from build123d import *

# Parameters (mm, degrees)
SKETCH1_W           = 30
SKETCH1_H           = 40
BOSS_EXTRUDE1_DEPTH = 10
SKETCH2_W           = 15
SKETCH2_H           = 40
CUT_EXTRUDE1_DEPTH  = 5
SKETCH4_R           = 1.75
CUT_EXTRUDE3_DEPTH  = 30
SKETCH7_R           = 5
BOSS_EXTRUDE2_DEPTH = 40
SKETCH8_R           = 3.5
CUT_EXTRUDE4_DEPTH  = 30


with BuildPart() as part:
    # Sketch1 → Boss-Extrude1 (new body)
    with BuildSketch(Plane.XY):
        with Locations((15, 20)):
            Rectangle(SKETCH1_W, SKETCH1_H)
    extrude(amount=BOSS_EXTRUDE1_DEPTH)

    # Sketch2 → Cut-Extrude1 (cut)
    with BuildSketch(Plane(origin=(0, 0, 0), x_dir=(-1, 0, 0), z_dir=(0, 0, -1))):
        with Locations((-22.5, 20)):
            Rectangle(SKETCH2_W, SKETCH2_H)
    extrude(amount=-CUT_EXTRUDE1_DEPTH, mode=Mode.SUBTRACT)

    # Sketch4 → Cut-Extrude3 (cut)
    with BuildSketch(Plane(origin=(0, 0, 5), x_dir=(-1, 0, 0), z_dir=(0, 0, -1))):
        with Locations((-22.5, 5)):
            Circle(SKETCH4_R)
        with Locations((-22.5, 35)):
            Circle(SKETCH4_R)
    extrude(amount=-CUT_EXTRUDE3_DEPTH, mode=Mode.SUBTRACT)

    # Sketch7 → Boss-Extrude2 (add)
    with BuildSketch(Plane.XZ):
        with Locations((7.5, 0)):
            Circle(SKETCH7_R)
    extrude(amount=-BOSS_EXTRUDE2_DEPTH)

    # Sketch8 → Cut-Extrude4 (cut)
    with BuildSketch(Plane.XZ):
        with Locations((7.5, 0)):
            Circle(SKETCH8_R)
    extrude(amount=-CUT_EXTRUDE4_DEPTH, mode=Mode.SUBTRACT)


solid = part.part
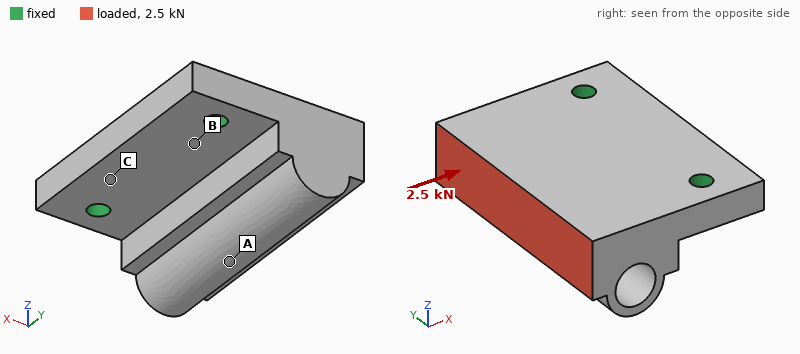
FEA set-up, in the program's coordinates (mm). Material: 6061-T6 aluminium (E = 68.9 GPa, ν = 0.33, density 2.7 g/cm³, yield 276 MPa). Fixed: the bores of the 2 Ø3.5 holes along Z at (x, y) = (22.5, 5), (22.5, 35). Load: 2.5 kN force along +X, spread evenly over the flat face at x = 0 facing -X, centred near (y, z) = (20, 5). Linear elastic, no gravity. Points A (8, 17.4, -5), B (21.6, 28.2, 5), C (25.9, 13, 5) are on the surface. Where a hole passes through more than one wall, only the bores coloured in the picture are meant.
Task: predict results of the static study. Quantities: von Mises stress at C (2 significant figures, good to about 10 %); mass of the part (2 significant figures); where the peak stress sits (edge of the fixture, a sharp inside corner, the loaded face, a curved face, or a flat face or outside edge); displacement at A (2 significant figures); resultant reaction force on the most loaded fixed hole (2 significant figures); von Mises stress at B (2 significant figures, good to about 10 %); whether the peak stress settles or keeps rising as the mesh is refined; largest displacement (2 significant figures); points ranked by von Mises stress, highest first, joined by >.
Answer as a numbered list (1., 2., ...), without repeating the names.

1. 16 MPa
2. 25 g
3. edge of the fixture
4. 44 µm
5. 1.3 kN
6. 28 MPa
7. keeps rising
8. 52 µm
9. B > C > A
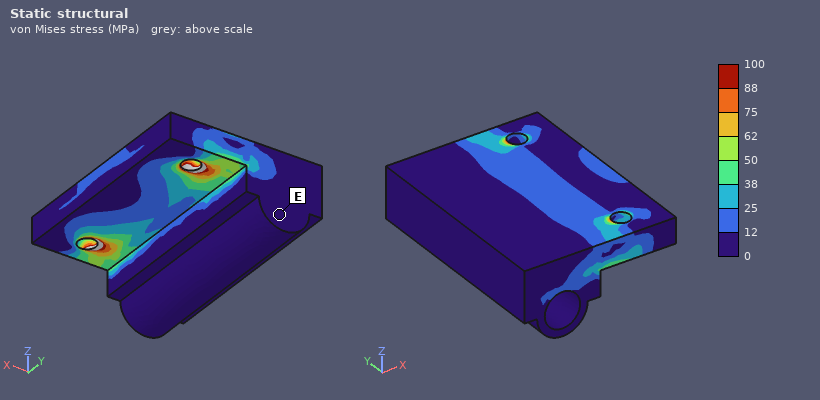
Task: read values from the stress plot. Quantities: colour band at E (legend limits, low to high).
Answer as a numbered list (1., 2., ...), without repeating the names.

1. 0 to 12 MPa
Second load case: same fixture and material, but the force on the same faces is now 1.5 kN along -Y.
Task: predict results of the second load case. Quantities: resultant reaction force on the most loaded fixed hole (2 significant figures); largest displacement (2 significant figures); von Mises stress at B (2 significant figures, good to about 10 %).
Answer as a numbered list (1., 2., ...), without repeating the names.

1. 1.3 kN
2. 12 µm
3. 13 MPa
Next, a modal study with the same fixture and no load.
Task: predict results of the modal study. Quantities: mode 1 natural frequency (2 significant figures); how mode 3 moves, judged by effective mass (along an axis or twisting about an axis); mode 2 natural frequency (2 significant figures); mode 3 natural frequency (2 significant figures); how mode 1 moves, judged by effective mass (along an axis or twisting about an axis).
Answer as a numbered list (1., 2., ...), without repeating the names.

1. 4600 Hz
2. along Y
3. 13 kHz
4. 19 kHz
5. along Z
